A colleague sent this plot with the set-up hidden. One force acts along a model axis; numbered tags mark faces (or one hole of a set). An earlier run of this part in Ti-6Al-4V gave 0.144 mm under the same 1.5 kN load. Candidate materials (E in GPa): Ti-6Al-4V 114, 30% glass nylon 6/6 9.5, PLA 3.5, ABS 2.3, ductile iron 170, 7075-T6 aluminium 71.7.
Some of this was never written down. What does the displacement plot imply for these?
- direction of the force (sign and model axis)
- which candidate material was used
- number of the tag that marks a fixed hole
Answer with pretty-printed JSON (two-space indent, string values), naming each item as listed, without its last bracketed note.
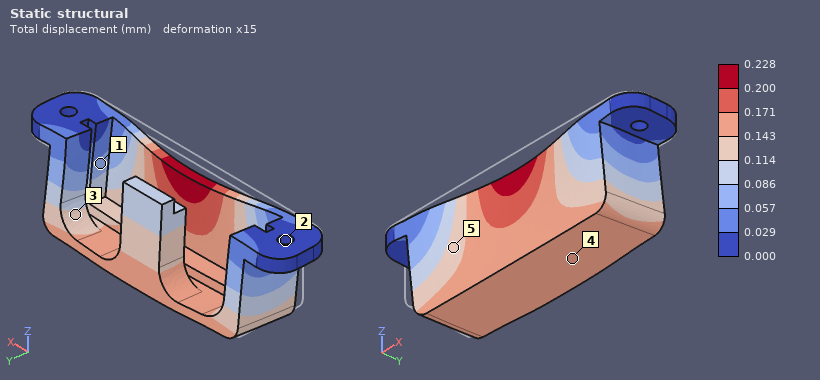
{
  "direction of the force": "+Y",
  "which candidate material was used": "7075-T6 aluminium",
  "number of the tag that marks a fixed hole": "2"
}
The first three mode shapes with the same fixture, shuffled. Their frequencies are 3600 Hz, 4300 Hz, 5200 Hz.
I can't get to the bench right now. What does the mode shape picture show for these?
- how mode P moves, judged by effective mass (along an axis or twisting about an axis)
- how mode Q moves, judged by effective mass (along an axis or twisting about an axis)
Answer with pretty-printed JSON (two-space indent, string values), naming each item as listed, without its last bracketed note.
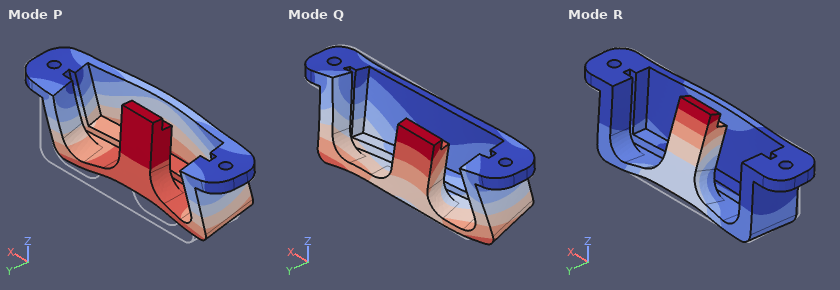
{
  "how mode P moves, judged by effective mass": "along Y",
  "how mode Q moves, judged by effective mass": "along X"
}
